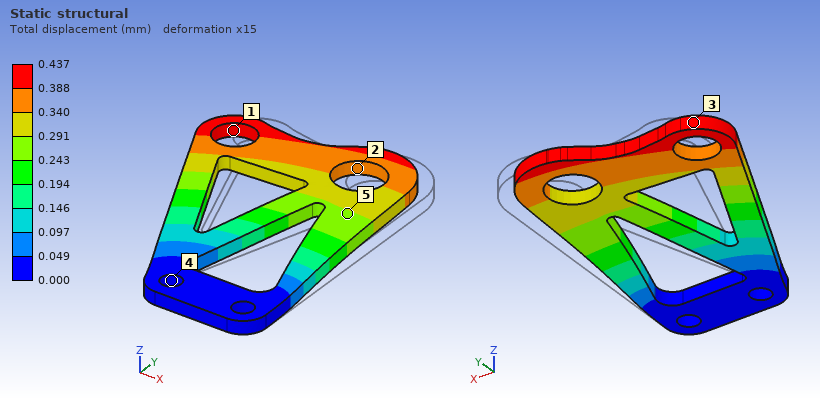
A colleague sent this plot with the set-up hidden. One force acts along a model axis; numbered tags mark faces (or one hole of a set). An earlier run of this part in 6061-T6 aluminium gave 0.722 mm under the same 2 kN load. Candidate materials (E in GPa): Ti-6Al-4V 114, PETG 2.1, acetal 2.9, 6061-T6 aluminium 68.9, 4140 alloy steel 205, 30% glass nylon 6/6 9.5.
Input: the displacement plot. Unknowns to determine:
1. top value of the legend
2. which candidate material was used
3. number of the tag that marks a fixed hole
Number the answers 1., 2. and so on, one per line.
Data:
1. 0.437 mm
2. Ti-6Al-4V
3. 4
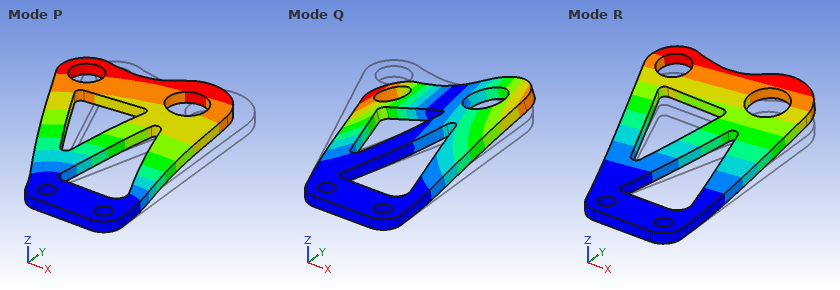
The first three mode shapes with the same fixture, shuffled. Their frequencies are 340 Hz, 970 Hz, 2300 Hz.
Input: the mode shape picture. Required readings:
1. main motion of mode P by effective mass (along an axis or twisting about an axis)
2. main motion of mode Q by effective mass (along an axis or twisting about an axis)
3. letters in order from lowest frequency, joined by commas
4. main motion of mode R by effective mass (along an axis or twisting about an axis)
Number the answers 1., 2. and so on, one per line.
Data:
1. along X
2. twisting about Y
3. R, Q, P
4. along Z
